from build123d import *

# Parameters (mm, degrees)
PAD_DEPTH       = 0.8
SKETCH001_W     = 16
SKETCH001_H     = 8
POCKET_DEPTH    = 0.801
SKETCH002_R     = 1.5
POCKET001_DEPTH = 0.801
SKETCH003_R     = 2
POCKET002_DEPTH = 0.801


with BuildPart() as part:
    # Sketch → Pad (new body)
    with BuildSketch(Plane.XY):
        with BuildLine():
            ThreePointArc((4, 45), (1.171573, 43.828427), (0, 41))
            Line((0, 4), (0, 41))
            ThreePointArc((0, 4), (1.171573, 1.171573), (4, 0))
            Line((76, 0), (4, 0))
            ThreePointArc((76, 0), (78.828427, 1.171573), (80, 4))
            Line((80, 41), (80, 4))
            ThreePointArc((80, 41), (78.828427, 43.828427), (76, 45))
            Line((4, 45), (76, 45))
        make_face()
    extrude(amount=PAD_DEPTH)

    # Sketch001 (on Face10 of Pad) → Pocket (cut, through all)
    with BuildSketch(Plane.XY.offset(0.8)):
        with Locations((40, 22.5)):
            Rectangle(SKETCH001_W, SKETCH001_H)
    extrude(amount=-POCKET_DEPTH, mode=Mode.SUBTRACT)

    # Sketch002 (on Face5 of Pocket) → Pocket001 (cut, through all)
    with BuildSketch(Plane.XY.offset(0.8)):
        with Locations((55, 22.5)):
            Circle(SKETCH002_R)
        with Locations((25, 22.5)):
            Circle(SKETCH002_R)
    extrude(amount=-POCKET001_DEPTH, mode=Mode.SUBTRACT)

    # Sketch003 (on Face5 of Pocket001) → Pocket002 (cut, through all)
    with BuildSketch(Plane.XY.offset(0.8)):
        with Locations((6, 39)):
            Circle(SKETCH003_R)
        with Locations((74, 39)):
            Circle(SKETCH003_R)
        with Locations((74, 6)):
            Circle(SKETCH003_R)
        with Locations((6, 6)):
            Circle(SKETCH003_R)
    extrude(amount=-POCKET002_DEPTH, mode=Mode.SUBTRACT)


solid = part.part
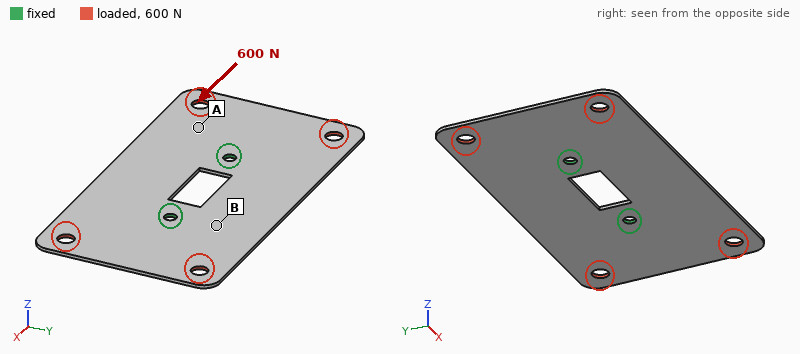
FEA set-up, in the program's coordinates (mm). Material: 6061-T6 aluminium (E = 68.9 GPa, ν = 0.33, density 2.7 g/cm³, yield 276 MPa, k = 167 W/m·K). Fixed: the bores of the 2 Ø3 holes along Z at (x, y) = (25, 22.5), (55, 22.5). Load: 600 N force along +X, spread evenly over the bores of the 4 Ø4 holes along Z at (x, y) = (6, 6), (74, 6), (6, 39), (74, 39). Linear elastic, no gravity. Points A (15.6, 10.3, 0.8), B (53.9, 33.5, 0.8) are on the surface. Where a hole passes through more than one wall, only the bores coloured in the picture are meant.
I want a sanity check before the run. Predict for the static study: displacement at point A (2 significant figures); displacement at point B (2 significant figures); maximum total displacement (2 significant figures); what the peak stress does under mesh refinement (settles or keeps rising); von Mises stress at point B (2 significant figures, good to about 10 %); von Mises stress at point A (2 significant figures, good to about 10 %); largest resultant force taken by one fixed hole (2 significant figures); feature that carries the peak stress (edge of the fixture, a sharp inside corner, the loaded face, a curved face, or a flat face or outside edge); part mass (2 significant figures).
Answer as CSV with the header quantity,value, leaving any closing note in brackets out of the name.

quantity,value
displacement at point A,5.0 µm
displacement at point B,4.1 µm
maximum total displacement,9.2 µm
what the peak stress does under mesh refinement,keeps rising
von Mises stress at point B,5.7 MPa
von Mises stress at point A,11 MPa
largest resultant force taken by one fixed hole,300 N
feature that carries the peak stress,edge of the fixture
part mass,7.3 g
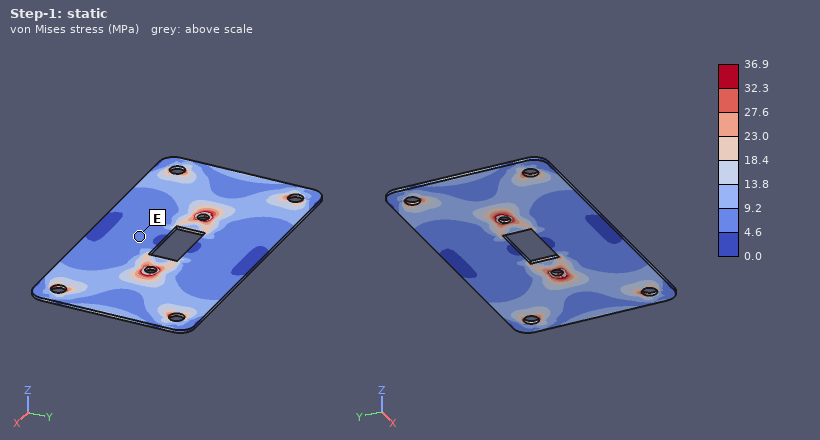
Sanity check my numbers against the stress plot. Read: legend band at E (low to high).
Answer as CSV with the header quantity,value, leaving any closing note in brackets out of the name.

quantity,value
legend band at E,4.6 to 9.2 MPa
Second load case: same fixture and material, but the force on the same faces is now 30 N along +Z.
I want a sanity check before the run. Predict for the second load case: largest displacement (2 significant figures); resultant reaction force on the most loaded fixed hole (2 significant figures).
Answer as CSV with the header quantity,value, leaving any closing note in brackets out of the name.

quantity,value
largest displacement,0.58 mm
resultant reaction force on the most loaded fixed hole,15 N
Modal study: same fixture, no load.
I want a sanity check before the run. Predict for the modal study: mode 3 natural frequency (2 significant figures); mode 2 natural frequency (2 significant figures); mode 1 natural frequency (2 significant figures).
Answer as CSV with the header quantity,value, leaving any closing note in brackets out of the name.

quantity,value
mode 3 natural frequency,910 Hz
mode 2 natural frequency,900 Hz
mode 1 natural frequency,870 Hz
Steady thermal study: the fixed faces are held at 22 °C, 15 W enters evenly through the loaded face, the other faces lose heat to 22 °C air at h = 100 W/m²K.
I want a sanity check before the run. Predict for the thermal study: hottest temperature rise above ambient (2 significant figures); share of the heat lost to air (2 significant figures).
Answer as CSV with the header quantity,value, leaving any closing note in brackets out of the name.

quantity,value
hottest temperature rise above ambient,30 K
share of the heat lost to air,57 %
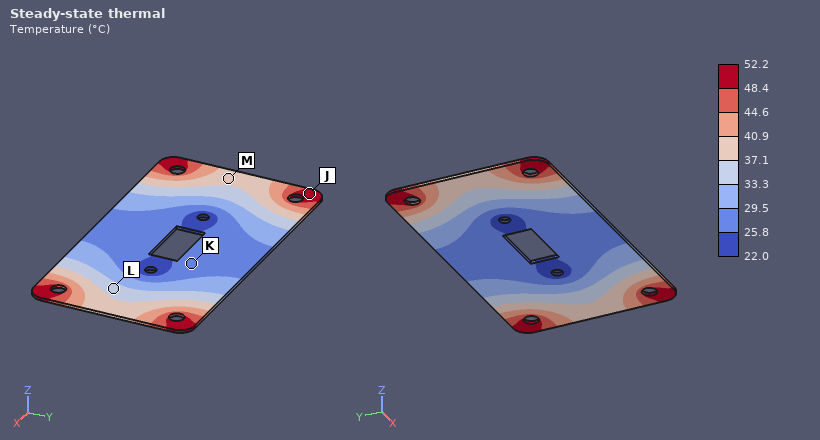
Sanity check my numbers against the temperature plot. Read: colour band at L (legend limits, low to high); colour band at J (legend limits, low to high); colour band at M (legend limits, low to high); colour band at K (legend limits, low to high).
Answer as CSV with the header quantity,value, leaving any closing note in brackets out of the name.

quantity,value
colour band at L,33.3 to 37.1 °C
colour band at J,48.4 to 52.2 °C
colour band at M,37.1 to 40.9 °C
colour band at K,25.8 to 29.5 °C
